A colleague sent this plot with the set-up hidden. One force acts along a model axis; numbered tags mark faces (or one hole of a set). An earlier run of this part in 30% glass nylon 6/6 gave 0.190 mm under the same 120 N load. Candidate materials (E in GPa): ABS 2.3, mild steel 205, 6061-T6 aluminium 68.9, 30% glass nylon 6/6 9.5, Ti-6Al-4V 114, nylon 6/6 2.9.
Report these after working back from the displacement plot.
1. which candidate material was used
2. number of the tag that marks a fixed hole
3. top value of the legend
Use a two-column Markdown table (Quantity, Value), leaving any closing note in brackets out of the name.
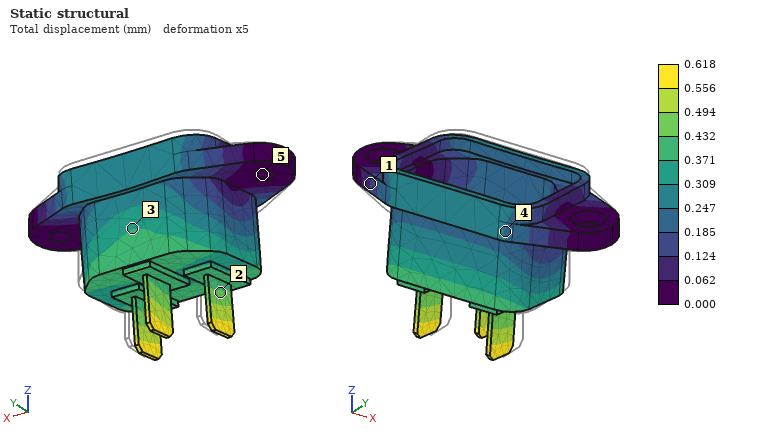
| Quantity | Value |
|---|---|
| which candidate material was used | nylon 6/6 |
| number of the tag that marks a fixed hole | 5 |
| top value of the legend | 0.618 mm |
